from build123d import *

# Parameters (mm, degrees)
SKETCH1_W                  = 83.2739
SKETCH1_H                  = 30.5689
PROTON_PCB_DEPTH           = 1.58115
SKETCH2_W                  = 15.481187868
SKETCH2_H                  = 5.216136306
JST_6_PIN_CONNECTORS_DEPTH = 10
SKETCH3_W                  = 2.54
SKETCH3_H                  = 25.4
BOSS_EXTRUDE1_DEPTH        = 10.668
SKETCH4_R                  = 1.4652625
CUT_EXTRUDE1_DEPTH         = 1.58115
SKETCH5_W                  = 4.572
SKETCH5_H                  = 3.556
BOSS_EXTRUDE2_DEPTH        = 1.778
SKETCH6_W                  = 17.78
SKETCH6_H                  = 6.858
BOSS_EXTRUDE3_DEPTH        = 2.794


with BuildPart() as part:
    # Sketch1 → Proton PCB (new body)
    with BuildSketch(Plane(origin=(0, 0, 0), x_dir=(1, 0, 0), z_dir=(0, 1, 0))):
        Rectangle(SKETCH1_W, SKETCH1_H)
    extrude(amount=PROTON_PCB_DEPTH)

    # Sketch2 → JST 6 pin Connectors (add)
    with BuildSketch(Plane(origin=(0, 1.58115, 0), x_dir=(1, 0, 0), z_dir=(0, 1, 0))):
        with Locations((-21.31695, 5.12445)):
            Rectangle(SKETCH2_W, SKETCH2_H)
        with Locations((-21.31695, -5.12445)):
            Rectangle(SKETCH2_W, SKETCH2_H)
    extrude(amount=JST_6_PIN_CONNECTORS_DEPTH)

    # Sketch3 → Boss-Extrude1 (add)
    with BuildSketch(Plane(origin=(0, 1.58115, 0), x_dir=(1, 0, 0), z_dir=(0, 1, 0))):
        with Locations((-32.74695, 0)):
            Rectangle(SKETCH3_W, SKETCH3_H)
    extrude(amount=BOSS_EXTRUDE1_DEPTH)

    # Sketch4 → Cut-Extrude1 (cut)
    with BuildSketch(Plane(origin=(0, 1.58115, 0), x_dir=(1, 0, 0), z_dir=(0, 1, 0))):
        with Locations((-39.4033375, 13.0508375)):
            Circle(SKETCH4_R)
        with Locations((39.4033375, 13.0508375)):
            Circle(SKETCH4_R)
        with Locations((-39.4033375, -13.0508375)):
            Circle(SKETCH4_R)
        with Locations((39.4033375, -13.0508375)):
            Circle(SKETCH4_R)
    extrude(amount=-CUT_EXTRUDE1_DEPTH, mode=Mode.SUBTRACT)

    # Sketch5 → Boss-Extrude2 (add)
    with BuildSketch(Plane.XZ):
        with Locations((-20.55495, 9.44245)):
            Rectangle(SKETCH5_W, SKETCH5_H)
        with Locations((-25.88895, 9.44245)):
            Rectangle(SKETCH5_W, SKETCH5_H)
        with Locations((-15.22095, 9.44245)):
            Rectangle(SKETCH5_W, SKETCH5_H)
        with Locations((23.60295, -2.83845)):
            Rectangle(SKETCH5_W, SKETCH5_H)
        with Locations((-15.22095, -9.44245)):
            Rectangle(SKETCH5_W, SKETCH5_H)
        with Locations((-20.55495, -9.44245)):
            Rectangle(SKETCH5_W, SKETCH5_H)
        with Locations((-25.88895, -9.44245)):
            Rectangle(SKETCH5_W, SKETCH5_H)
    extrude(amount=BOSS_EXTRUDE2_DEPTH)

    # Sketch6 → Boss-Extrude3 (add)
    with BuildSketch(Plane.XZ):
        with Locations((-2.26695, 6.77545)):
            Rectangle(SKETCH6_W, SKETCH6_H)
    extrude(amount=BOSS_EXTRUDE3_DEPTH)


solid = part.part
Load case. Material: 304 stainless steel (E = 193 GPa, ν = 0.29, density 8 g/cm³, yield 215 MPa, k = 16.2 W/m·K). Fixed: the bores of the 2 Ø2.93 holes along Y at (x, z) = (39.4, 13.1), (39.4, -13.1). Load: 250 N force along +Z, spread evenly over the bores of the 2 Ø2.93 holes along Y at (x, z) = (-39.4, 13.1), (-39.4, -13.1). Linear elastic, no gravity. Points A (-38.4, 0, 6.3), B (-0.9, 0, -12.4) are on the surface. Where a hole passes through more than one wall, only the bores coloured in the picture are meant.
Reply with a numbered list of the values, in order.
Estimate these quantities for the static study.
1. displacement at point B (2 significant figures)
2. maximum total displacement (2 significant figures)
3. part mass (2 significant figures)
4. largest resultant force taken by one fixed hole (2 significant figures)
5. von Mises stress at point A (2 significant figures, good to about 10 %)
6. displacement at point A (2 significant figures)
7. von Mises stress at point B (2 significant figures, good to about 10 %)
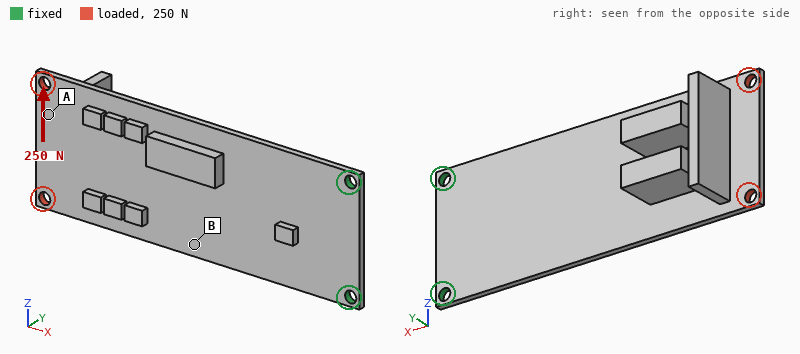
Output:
1. 24 µm
2. 69 µm
3. 55 g
4. 770 N
5. 10 MPa
6. 62 µm
7. 34 MPa
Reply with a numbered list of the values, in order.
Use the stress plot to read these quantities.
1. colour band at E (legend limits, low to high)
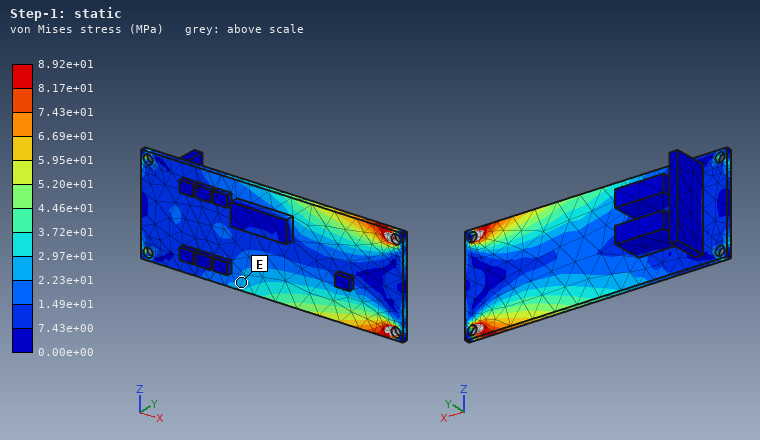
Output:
1. 2.23e+01 to 2.97e+01 MPa
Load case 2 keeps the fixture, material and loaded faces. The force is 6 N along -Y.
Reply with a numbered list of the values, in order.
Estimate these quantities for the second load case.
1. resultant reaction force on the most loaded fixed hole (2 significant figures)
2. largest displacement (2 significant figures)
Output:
1. 3.2 N
2. 0.48 mm
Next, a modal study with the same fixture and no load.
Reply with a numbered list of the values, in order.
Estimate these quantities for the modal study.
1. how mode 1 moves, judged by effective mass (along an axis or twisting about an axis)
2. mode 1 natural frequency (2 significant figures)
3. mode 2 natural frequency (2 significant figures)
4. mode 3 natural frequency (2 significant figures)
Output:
1. along Y
2. 130 Hz
3. 860 Hz
4. 1200 Hz
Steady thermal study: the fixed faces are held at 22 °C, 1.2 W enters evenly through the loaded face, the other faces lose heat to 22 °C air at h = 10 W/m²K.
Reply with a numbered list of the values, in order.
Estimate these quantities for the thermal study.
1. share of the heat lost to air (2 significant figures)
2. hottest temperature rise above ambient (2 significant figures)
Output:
1. 87 %
2. 52 K
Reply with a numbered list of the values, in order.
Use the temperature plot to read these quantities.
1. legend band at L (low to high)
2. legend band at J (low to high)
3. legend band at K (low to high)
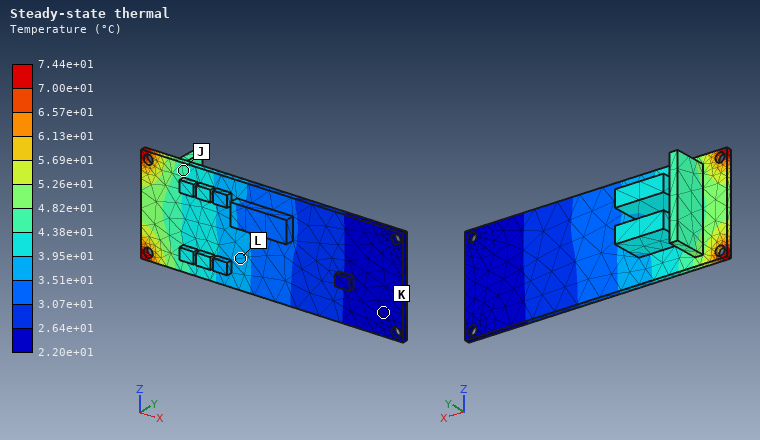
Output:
1. 3.51e+01 to 3.95e+01 °C
2. 4.38e+01 to 4.82e+01 °C
3. 2.20e+01 to 2.64e+01 °C
